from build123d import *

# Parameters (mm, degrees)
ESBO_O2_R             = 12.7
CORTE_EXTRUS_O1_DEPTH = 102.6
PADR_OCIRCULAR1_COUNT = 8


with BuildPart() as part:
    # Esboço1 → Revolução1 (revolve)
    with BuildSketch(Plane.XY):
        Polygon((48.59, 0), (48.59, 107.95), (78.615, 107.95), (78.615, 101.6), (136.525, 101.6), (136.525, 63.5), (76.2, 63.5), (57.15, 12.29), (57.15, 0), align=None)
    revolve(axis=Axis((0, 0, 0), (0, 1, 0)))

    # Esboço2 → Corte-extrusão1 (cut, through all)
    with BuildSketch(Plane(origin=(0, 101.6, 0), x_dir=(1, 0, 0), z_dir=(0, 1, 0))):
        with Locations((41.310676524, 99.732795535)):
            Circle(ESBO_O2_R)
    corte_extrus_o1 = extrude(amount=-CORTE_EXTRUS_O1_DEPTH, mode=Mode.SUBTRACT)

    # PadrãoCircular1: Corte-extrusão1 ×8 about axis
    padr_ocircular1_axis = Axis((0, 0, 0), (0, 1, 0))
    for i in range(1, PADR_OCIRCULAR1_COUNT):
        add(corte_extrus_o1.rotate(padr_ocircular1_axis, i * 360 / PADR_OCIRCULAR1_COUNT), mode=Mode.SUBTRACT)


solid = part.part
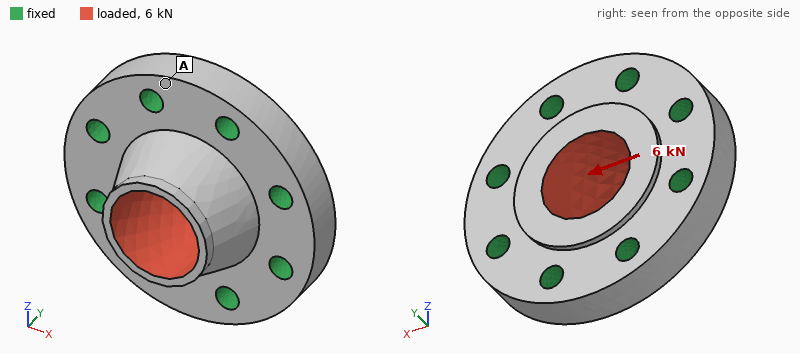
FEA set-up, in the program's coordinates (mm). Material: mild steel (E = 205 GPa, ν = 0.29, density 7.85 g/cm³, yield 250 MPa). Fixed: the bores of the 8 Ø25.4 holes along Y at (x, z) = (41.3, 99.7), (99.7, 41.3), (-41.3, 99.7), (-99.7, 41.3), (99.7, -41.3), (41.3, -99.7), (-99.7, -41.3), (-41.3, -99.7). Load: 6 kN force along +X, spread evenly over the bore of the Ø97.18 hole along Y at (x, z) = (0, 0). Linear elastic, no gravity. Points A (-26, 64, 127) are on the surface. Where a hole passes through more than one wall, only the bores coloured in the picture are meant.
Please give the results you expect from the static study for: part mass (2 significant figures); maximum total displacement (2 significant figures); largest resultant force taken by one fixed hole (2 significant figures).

18 kg
0.89 µm
1.1 kN
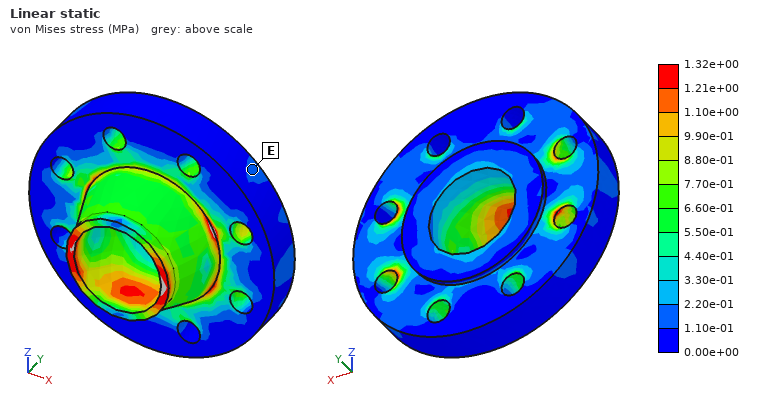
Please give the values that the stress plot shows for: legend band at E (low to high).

1.10e-01 to 2.20e-01 MPa
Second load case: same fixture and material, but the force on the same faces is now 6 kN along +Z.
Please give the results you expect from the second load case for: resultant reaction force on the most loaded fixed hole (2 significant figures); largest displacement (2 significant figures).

1.1 kN
0.89 µm
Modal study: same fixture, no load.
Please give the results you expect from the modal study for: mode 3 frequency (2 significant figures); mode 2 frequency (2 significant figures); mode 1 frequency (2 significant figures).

8300 Hz
8300 Hz
8100 Hz
